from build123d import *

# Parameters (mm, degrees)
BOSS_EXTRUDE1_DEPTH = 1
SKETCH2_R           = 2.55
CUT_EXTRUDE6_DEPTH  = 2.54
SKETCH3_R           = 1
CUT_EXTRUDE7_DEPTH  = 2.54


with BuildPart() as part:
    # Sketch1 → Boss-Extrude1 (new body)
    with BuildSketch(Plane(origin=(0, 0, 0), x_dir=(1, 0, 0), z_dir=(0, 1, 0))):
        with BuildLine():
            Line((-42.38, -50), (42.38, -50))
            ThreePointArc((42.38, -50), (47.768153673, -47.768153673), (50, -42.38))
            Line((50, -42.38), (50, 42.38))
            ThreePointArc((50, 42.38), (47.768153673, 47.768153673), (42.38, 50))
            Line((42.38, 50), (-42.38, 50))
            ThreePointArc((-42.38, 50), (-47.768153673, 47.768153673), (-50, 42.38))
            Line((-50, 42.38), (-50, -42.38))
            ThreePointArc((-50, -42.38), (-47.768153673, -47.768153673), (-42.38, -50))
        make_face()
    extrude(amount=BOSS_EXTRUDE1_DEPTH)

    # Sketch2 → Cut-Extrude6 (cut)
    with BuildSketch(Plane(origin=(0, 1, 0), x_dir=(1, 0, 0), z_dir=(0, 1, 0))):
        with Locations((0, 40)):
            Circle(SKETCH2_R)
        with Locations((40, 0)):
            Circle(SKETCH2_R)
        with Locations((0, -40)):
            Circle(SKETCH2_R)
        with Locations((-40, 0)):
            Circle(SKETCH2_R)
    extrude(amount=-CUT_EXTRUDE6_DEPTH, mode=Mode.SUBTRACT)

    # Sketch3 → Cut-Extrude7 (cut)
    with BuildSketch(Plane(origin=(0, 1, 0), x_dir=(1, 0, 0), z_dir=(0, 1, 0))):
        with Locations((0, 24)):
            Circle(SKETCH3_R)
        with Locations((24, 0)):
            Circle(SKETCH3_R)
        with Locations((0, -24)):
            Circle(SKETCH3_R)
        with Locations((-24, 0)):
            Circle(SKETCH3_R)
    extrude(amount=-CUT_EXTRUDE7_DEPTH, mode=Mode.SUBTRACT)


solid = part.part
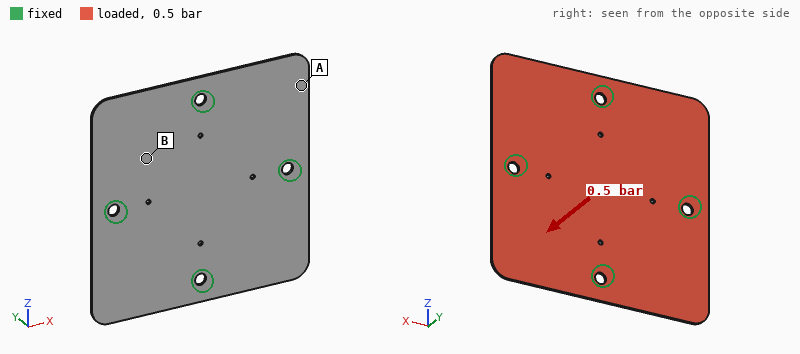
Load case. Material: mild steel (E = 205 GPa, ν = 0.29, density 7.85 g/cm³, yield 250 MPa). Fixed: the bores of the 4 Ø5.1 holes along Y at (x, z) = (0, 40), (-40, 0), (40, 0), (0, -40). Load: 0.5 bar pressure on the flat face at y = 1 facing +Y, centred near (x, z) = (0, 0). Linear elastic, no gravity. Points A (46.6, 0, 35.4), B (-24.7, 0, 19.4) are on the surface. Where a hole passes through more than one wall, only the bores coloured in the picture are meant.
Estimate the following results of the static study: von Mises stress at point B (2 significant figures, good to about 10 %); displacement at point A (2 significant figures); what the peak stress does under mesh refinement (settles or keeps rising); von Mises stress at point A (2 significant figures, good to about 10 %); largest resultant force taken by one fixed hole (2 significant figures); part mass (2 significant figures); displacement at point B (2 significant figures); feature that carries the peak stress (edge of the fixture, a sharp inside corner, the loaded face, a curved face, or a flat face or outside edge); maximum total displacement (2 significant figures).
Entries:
70 MPa
0.39 mm
keeps rising
44 MPa
120 N
77 g
0.11 mm
edge of the fixture
0.55 mm
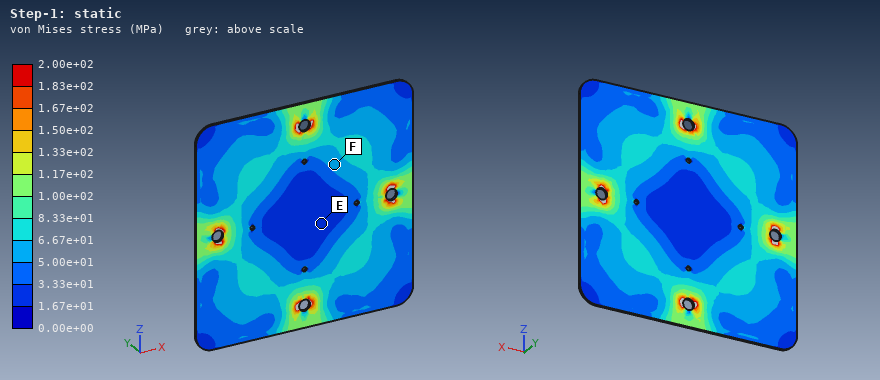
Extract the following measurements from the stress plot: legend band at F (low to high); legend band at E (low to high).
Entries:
5.00e+01 to 6.67e+01 MPa
1.67e+01 to 3.33e+01 MPa
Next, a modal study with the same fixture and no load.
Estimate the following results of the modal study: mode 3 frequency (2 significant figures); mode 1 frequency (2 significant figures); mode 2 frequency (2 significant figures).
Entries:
720 Hz
700 Hz
720 Hz
